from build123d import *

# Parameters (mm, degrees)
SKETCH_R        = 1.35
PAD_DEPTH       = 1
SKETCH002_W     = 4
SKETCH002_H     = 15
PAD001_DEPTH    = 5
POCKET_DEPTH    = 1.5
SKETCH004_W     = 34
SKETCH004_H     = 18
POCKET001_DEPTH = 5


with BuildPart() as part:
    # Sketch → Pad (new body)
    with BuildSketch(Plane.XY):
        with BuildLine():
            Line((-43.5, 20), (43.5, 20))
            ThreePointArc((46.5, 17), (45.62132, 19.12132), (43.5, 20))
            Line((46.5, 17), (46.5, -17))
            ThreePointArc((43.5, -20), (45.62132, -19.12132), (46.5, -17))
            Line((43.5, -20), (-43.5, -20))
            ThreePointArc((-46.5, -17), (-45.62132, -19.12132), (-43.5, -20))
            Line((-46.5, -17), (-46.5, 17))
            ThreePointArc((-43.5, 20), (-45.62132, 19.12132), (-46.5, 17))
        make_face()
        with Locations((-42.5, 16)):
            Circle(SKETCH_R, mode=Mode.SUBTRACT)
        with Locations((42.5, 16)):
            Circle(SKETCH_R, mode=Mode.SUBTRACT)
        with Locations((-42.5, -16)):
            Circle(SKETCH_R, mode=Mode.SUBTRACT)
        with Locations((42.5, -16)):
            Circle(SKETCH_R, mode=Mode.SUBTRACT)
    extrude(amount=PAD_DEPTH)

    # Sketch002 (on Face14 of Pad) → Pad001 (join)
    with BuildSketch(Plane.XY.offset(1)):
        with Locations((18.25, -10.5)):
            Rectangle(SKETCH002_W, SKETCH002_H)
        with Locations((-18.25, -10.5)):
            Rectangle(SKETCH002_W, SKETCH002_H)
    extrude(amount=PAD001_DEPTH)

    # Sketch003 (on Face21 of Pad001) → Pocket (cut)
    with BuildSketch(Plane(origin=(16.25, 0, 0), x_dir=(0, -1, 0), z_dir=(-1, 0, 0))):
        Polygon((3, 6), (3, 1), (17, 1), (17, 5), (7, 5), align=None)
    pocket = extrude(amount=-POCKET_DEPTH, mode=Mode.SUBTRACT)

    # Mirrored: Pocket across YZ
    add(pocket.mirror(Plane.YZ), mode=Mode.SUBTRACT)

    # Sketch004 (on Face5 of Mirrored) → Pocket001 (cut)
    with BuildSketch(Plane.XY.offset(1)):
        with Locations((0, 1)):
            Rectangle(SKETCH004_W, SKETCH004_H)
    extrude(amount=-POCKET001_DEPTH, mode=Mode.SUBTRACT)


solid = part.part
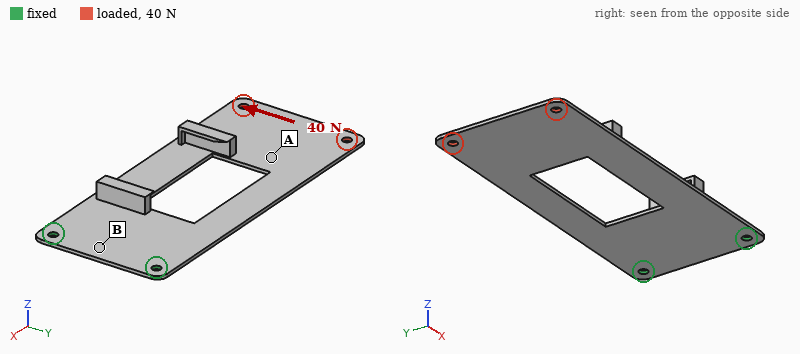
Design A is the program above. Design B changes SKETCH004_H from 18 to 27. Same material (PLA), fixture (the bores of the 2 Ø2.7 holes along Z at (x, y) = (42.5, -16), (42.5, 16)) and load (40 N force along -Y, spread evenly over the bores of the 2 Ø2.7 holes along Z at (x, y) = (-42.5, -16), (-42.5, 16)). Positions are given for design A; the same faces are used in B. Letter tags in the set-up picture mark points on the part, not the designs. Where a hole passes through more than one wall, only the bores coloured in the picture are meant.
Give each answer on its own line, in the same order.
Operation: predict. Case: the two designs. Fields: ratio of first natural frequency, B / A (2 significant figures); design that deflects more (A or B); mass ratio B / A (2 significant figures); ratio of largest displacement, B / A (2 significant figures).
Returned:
0.90
B
0.91
2.1
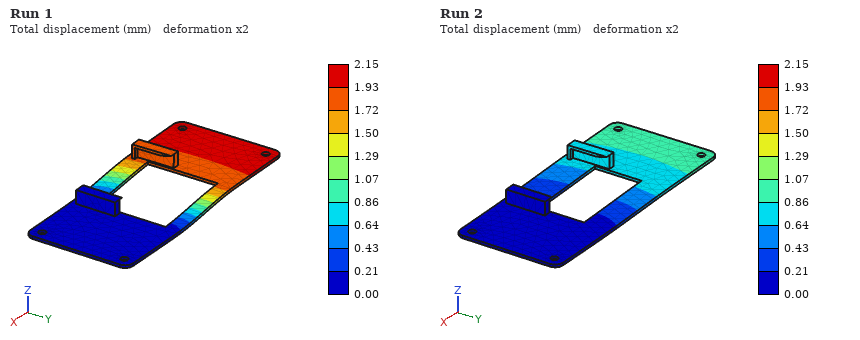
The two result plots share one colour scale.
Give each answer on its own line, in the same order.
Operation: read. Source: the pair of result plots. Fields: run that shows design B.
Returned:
Run 1
